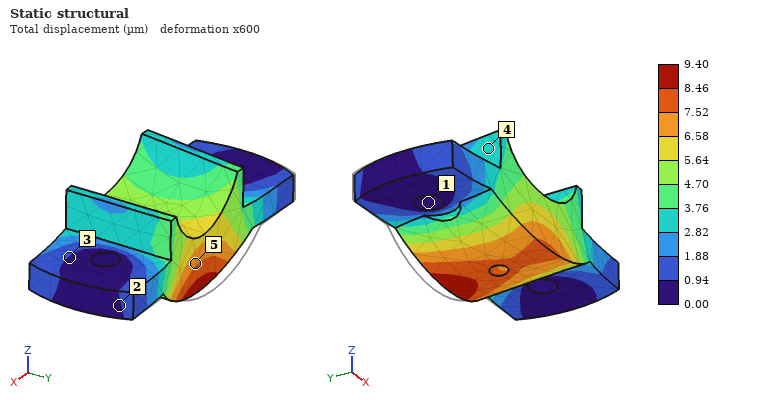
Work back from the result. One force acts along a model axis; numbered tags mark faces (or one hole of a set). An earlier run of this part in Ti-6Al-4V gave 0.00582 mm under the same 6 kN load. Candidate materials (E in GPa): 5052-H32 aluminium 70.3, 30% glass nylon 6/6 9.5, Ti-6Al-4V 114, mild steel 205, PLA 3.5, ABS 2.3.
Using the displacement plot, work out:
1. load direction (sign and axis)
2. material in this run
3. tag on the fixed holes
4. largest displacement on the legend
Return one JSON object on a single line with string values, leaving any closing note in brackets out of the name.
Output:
{"load direction": "-Y", "material in this run": "5052-H32 aluminium", "tag on the fixed holes": "1", "largest displacement on the legend": "9.40 µm"}
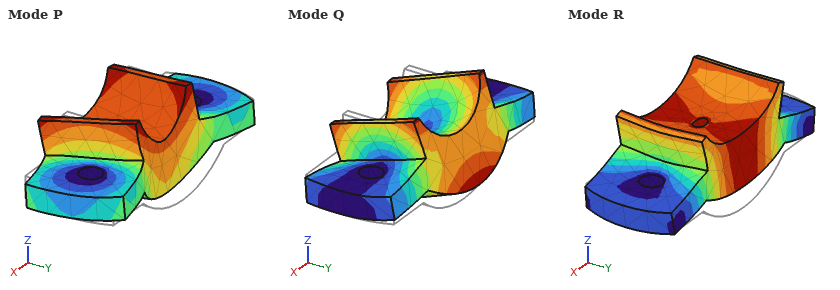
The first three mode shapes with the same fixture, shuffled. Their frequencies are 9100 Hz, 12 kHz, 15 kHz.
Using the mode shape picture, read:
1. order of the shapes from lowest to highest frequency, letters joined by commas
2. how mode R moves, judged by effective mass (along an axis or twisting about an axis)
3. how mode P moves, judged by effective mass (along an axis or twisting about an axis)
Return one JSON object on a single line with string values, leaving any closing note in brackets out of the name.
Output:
{"order of the shapes from lowest to highest frequency, letters joined by commas": "Q, R, P", "how mode R moves, judged by effective mass": "along Z", "how mode P moves, judged by effective mass": "along Y"}
